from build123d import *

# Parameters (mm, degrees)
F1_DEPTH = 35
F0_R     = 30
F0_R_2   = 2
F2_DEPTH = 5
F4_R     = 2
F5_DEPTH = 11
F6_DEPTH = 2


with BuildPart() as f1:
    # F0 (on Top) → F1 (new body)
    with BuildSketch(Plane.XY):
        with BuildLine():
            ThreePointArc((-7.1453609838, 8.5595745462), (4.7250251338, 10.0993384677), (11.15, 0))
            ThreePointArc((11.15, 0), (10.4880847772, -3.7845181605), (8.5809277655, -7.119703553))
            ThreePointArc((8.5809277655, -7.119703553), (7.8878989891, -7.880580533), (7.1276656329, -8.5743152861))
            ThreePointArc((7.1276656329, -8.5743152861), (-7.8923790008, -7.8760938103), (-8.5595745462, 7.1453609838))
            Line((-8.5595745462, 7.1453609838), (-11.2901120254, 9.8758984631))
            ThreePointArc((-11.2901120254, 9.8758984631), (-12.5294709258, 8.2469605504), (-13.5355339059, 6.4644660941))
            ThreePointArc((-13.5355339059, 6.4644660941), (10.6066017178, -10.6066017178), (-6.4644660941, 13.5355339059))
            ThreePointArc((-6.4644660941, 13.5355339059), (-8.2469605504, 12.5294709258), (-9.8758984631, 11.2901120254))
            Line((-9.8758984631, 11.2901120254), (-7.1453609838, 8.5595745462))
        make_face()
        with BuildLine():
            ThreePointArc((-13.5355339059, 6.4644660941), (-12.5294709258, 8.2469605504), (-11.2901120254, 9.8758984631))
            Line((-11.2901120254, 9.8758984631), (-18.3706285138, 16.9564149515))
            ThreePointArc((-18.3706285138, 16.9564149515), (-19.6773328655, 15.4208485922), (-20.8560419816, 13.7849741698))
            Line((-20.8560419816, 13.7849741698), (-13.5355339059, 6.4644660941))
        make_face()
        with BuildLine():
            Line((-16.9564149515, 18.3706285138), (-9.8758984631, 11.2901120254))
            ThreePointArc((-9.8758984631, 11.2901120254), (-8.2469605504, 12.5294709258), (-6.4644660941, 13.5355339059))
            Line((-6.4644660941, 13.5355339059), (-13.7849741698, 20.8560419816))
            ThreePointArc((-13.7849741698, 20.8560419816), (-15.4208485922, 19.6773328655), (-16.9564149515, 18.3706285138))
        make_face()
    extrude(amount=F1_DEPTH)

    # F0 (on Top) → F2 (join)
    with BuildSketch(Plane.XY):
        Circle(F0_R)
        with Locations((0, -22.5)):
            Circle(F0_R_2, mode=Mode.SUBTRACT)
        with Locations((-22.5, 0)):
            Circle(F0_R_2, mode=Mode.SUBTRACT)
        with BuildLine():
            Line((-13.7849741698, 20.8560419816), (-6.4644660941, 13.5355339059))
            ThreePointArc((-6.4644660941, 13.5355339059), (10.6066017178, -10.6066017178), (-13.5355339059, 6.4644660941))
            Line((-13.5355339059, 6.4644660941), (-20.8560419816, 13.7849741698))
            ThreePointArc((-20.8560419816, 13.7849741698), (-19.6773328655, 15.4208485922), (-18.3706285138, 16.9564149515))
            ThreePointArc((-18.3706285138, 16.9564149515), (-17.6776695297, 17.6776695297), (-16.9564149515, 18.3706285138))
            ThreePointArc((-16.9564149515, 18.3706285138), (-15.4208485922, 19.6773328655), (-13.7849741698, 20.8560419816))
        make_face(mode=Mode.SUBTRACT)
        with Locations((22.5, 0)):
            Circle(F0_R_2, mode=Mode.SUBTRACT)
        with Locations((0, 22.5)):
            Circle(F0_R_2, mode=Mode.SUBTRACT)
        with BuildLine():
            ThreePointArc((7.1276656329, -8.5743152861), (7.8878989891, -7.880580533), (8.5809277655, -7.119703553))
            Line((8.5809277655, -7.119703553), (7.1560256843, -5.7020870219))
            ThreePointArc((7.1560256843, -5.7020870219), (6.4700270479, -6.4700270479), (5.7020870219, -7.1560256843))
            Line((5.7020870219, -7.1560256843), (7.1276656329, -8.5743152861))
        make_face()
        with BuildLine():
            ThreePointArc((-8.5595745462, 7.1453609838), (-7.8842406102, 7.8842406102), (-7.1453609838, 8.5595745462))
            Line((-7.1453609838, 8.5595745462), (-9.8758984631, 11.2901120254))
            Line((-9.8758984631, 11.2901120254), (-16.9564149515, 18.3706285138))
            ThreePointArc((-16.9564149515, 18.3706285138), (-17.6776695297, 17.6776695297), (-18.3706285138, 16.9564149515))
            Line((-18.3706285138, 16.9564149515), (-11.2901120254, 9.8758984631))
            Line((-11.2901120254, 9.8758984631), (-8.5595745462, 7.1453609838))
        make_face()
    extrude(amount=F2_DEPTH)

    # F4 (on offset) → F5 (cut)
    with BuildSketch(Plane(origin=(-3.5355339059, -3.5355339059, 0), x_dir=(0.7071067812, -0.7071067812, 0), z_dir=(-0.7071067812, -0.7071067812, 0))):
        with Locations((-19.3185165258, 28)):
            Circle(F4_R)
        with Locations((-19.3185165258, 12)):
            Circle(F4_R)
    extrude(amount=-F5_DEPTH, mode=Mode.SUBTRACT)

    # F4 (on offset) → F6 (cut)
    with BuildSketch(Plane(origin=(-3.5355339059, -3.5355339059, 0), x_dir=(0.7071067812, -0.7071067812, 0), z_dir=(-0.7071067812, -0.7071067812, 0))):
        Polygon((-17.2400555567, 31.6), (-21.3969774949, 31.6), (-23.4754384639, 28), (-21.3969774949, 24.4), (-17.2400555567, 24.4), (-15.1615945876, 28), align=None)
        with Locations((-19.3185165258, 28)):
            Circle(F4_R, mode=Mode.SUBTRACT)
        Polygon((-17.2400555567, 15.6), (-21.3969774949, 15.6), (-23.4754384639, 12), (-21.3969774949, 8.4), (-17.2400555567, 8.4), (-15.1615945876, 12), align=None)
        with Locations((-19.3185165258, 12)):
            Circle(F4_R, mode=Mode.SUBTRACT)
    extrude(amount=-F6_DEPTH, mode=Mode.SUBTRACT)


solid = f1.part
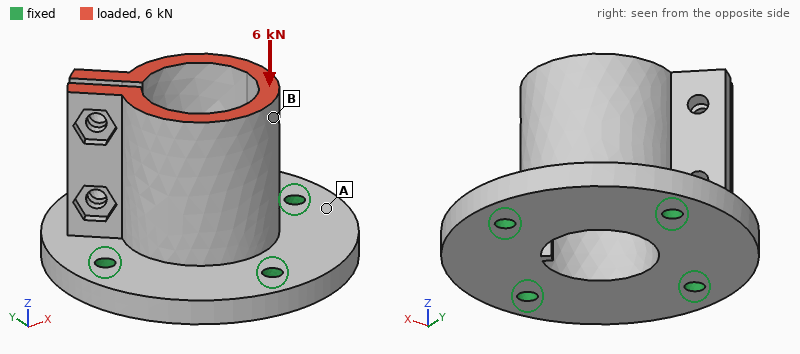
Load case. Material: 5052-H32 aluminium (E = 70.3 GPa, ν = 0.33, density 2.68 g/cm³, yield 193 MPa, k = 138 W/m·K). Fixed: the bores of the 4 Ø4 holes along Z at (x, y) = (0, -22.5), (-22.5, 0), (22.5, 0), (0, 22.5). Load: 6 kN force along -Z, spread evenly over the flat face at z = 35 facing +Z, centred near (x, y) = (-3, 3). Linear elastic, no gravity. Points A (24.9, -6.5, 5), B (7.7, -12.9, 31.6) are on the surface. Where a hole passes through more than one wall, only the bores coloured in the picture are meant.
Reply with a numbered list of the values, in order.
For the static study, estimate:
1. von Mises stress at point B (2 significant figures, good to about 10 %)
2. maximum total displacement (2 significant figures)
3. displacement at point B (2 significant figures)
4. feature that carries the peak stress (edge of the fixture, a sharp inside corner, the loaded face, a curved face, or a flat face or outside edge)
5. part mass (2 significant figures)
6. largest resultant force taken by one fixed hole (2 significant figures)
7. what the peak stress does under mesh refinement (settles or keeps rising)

1. 22 MPa
2. 54 µm
3. 21 µm
4. edge of the fixture
5. 62 g
6. 1.9 kN
7. keeps rising
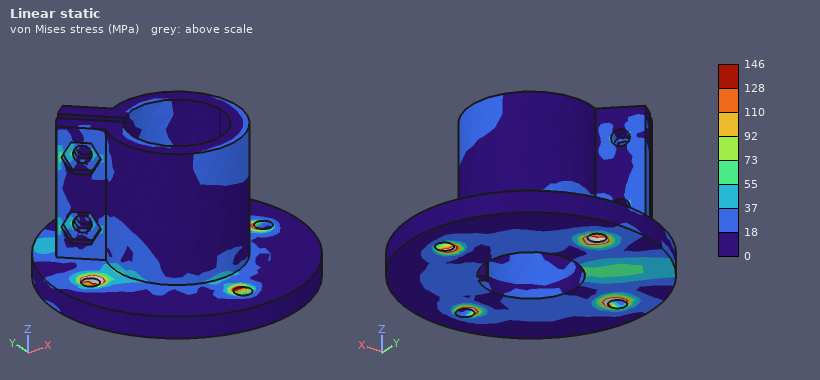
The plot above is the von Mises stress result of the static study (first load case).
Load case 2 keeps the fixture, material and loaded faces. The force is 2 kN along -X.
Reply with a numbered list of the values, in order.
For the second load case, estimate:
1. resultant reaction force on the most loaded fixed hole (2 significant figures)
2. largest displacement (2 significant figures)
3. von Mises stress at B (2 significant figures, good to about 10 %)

1. 1.7 kN
2. 0.23 mm
3. 25 MPa
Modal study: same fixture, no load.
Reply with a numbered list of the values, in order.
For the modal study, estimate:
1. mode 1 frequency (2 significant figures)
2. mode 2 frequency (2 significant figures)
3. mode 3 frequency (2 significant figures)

1. 5200 Hz
2. 6400 Hz
3. 8500 Hz
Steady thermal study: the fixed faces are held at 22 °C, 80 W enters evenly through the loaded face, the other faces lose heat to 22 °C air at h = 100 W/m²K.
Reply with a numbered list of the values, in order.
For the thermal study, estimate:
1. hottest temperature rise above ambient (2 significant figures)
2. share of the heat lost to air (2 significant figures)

1. 55 K
2. 28 %
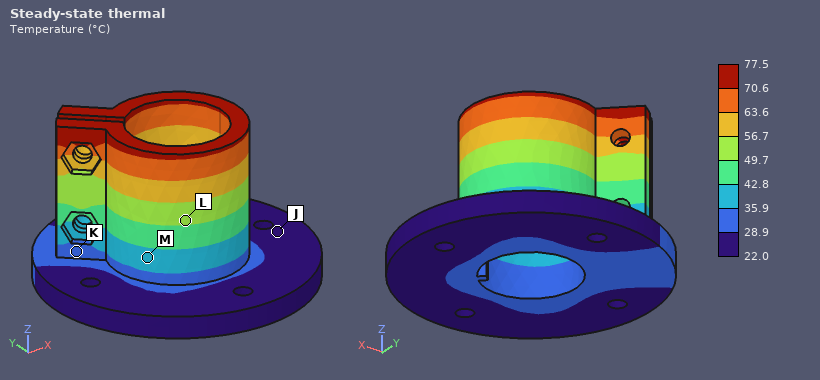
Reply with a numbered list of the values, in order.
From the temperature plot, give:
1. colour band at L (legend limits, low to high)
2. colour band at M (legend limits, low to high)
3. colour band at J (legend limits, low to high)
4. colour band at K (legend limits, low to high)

1. 49.7 to 56.7 °C
2. 35.9 to 42.8 °C
3. 22.0 to 28.9 °C
4. 28.9 to 35.9 °C
